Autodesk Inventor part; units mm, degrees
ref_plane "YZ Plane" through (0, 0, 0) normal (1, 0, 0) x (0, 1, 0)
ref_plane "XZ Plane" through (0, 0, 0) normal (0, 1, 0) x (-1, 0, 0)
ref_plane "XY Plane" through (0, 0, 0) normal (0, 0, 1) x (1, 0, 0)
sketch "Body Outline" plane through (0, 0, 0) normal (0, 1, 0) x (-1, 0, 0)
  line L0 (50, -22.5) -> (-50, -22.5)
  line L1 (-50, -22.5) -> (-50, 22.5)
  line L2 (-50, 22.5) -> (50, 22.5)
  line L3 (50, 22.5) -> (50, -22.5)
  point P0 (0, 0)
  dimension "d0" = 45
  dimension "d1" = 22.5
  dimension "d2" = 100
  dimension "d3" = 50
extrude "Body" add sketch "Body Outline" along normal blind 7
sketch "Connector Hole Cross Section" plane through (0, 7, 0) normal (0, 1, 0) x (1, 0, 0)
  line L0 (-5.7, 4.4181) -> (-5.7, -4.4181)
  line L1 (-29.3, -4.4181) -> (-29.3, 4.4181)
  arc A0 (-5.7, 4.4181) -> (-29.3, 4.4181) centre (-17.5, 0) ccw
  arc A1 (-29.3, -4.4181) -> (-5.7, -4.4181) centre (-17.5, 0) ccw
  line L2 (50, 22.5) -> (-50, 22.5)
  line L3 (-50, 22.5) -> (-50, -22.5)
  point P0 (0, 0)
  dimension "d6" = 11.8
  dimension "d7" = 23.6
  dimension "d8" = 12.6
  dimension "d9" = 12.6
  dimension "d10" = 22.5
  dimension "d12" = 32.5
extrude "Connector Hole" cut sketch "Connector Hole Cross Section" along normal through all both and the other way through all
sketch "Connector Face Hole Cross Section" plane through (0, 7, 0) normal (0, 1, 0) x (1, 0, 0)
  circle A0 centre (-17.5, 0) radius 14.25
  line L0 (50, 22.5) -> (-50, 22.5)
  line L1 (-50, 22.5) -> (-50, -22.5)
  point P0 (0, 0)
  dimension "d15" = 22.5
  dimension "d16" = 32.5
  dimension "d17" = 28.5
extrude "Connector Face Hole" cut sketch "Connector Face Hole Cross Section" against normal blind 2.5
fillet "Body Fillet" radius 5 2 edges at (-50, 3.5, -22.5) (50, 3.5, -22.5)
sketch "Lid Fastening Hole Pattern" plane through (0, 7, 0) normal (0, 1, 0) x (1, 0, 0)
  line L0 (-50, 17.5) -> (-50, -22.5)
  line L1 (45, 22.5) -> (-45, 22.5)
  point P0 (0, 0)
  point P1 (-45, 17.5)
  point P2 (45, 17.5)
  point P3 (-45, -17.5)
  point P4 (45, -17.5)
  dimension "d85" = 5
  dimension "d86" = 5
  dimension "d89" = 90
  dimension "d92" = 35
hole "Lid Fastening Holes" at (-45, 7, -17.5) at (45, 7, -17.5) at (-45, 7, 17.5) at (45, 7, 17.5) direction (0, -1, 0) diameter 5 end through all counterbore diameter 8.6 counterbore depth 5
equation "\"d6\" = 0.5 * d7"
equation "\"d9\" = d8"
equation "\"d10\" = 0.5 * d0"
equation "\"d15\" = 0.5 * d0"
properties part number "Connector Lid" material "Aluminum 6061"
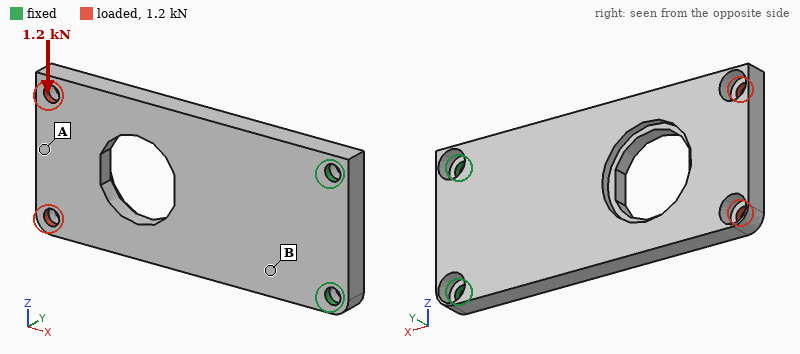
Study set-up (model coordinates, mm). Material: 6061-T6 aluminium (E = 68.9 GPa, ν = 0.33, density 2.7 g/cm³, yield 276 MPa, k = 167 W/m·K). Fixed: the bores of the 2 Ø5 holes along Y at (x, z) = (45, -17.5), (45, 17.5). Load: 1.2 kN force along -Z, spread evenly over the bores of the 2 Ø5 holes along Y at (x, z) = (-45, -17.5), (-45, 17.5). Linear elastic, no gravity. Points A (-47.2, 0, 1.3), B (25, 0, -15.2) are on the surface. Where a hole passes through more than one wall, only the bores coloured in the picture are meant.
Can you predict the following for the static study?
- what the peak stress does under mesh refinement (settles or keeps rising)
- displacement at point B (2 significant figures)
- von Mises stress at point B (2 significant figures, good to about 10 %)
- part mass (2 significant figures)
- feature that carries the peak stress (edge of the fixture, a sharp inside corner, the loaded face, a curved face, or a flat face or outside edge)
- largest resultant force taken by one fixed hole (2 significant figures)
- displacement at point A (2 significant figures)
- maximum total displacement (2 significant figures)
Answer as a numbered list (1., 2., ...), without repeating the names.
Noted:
1. keeps rising
2. 0.038 mm
3. 39 MPa
4. 71 g
5. edge of the fixture
6. 3.0 kN
7. 0.19 mm
8. 0.22 mm
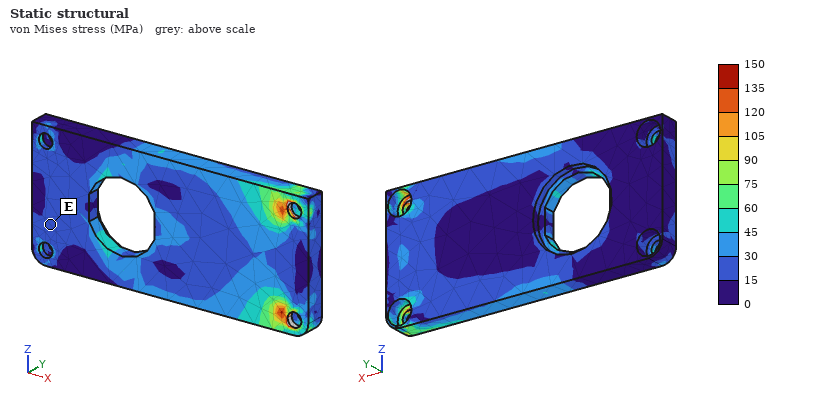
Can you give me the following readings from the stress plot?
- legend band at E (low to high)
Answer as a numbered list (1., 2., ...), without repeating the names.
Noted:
1. 15 to 30 MPa
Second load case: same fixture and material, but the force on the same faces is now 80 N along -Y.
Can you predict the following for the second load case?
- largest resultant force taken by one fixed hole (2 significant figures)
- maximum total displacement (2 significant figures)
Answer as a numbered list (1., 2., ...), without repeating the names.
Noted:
1. 43 N
2. 0.55 mm
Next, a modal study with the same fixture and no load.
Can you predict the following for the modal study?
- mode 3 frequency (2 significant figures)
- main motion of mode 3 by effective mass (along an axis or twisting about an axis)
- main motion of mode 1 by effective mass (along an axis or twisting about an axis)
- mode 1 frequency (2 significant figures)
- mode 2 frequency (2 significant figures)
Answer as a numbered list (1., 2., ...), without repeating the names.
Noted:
1. 2800 Hz
2. along Y
3. along Y
4. 450 Hz
5. 2400 Hz
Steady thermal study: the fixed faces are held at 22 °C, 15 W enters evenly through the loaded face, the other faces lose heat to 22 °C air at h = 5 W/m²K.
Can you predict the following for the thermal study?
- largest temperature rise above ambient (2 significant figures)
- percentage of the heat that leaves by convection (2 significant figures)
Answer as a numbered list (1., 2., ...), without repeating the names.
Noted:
1. 44 K
2. 6.8 %
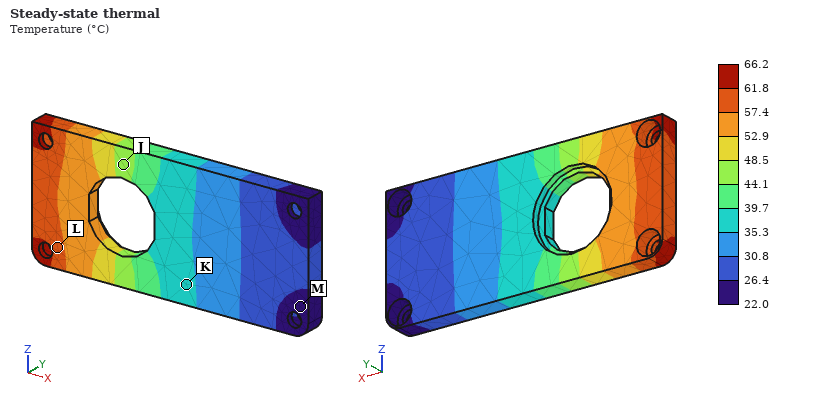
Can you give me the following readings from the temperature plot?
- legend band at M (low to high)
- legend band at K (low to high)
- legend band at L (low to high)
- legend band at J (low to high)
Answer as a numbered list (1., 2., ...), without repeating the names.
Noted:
1. 22.0 to 26.4 °C
2. 35.3 to 39.7 °C
3. 57.4 to 61.8 °C
4. 44.1 to 48.5 °C
